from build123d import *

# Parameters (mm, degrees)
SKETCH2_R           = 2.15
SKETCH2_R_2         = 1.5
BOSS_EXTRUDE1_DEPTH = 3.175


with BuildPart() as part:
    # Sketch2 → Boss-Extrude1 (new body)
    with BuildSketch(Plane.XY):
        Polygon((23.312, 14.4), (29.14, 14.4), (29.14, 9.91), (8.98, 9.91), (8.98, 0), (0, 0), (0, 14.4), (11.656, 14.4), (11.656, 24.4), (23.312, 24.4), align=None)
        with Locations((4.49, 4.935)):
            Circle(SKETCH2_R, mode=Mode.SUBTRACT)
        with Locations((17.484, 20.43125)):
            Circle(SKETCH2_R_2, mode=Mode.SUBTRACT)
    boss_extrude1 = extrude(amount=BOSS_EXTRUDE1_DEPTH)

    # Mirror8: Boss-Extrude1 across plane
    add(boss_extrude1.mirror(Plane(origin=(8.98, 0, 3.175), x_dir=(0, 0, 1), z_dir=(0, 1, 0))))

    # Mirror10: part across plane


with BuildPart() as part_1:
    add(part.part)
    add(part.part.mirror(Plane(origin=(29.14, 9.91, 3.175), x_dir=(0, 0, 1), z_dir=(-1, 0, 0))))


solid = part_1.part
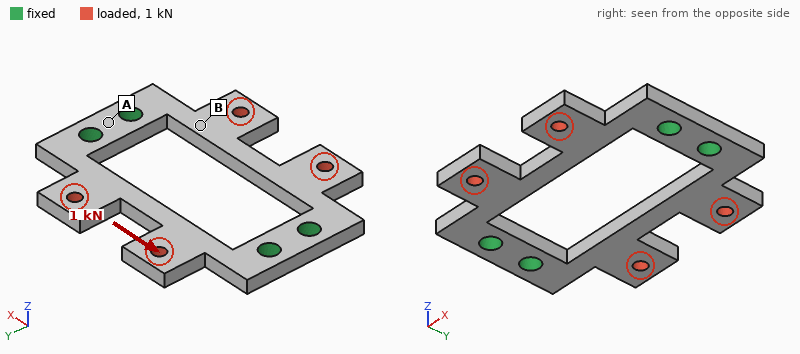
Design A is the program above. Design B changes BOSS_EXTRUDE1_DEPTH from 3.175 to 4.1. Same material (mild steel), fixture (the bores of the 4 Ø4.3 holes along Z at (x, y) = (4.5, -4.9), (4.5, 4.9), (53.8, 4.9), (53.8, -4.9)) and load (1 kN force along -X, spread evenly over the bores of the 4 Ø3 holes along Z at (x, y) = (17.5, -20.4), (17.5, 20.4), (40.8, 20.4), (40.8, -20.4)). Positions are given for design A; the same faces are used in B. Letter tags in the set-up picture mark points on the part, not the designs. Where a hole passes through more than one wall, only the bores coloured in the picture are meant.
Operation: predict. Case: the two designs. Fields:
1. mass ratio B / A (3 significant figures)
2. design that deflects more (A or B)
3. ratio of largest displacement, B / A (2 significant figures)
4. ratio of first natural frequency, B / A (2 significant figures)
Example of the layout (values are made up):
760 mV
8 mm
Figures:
1.29
A
0.76
1.3
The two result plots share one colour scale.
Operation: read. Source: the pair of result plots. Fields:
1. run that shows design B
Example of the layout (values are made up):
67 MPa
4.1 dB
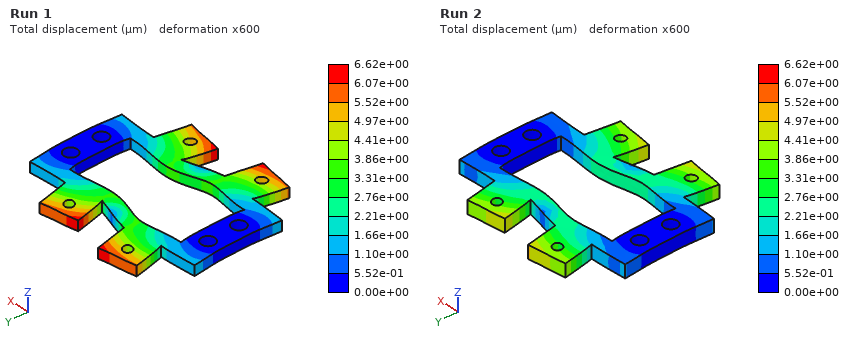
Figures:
Run 2
